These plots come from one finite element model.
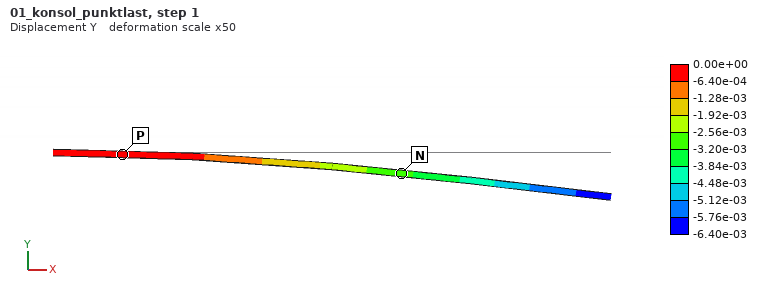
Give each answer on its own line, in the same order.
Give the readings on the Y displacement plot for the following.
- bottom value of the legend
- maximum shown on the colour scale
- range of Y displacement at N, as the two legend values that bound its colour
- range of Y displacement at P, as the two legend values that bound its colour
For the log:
-6.40e-03
0.00e+00
-3.20e-03 to -2.56e-03
-6.40e-04 to 0.00e+00
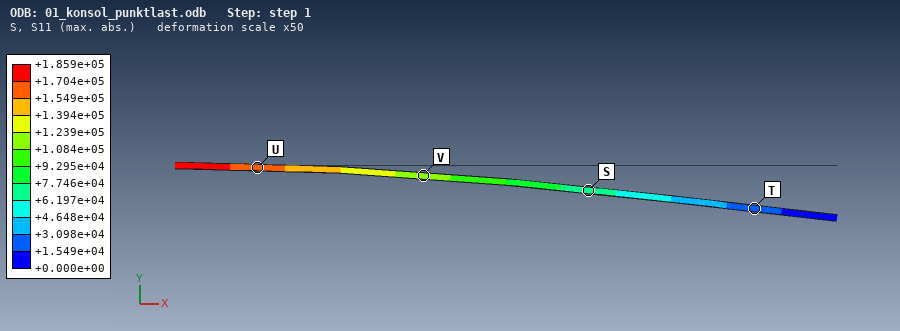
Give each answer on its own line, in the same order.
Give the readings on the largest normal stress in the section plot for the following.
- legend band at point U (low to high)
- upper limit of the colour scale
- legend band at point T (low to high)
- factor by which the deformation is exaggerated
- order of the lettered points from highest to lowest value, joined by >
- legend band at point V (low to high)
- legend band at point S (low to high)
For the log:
+1.549e+05 to +1.704e+05
+1.859e+05
+1.549e+04 to +3.098e+04
50
U > V > S > T
+1.084e+05 to +1.239e+05
+6.197e+04 to +7.746e+04
